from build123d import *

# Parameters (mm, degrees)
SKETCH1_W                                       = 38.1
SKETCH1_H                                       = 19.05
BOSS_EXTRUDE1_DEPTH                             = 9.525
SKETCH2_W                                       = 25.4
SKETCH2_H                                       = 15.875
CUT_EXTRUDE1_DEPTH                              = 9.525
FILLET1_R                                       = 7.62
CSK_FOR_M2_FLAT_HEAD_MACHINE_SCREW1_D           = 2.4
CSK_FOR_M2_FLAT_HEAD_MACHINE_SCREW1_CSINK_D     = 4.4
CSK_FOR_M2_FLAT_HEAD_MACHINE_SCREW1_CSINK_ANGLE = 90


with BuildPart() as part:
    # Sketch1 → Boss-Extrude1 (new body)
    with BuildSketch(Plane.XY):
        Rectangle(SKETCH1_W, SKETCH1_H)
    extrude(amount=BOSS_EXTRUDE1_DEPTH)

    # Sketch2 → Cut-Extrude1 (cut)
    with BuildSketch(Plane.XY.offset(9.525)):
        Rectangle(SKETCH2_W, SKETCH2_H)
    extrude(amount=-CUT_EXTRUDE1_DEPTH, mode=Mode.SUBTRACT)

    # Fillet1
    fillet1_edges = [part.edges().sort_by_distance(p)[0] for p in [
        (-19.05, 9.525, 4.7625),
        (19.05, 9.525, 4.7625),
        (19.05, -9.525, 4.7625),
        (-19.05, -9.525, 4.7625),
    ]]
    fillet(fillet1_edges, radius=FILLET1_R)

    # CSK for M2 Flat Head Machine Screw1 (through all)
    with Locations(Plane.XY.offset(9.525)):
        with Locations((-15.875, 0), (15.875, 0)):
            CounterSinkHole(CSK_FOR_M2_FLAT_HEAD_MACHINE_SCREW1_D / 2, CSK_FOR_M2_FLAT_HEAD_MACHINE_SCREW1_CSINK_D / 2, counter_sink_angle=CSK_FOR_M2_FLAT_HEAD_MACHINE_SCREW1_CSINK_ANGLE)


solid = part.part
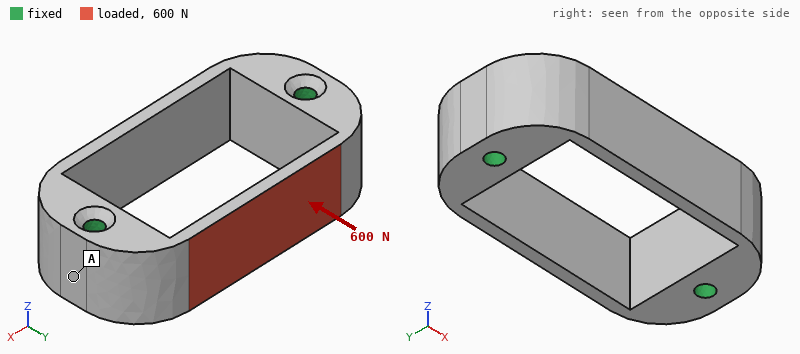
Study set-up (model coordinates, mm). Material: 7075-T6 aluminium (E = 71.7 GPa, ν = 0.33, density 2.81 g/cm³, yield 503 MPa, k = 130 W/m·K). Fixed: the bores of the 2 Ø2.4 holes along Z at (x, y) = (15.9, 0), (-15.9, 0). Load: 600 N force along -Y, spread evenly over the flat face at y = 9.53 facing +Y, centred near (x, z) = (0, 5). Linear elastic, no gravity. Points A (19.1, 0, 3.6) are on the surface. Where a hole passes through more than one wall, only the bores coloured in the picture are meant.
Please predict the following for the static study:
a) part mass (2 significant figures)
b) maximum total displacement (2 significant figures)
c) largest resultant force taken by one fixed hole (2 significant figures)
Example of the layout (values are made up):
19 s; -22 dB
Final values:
7.0 g; 0.18 mm; 420 N
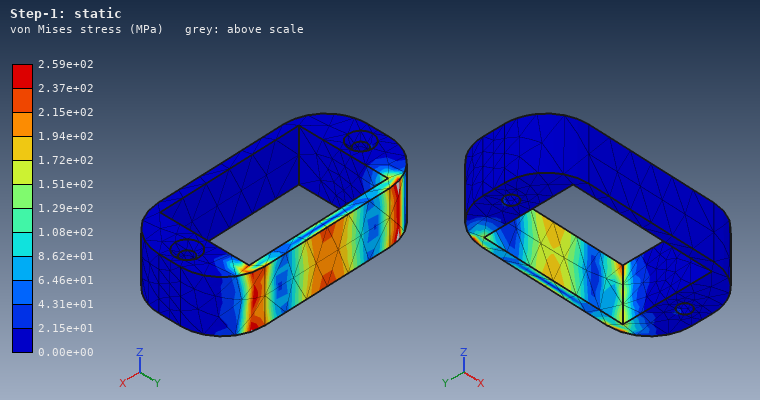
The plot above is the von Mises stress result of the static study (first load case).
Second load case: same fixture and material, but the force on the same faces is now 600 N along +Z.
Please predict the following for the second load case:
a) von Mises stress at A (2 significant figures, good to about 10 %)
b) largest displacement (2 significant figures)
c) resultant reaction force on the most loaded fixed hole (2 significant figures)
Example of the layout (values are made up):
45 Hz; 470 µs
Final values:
13 MPa; 34 µm; 300 N
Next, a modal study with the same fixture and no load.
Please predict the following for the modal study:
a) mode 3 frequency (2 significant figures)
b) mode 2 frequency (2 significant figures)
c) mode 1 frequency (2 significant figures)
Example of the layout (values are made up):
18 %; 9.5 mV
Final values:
21 kHz; 11 kHz; 11 kHz
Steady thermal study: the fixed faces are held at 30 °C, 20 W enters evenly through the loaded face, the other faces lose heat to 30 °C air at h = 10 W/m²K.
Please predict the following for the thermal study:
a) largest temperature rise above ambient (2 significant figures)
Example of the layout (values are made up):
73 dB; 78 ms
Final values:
54 K
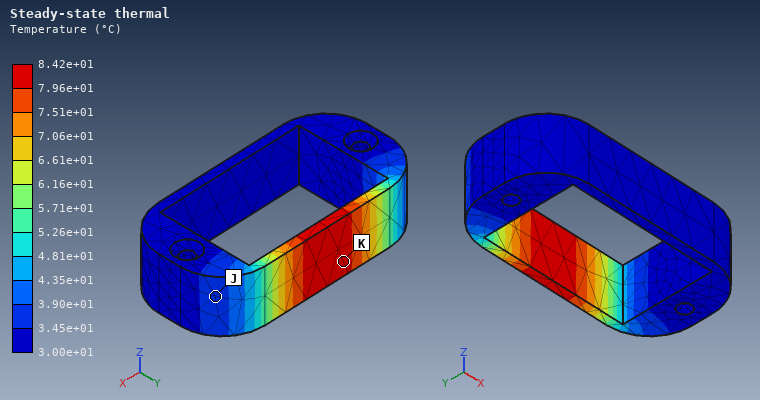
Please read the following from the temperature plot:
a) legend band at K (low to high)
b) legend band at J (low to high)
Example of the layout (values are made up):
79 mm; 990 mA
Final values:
7.96e+01 to 8.42e+01 °C; 3.45e+01 to 3.90e+01 °C
